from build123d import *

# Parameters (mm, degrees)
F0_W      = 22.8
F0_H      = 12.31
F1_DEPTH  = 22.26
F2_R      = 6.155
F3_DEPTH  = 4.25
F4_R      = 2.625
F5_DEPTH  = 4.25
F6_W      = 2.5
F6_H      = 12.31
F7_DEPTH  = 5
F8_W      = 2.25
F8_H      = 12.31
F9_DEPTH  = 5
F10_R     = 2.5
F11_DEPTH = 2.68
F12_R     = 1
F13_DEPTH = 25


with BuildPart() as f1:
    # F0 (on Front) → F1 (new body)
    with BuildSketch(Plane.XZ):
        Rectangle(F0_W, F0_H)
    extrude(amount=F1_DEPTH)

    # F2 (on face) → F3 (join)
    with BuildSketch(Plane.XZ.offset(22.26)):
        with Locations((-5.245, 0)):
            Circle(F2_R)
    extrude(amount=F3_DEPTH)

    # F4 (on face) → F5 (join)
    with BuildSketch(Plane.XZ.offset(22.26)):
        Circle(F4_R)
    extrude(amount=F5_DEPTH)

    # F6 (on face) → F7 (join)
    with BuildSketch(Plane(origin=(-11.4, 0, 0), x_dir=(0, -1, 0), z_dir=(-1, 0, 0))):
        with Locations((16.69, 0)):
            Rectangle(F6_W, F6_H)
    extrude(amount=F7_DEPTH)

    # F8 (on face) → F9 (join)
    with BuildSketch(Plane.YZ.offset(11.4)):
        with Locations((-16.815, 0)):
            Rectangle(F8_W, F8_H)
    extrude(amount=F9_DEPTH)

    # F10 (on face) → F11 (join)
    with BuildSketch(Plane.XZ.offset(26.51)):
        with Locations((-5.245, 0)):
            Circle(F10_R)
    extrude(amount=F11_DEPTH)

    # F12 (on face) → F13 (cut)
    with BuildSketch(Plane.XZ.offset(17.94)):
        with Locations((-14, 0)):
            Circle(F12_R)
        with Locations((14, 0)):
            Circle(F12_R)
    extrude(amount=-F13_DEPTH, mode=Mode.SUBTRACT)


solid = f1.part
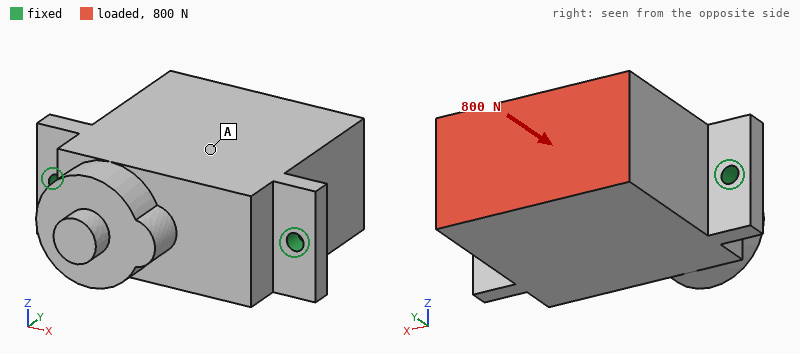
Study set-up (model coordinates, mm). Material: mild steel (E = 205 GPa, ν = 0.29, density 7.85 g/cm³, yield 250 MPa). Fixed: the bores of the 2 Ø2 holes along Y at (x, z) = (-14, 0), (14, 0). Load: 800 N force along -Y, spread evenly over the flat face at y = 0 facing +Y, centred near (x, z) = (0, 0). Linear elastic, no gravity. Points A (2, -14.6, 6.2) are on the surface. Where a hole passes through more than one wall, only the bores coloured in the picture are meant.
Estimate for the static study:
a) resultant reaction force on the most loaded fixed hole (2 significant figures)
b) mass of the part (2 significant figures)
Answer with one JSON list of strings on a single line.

["400 N", "56 g"]
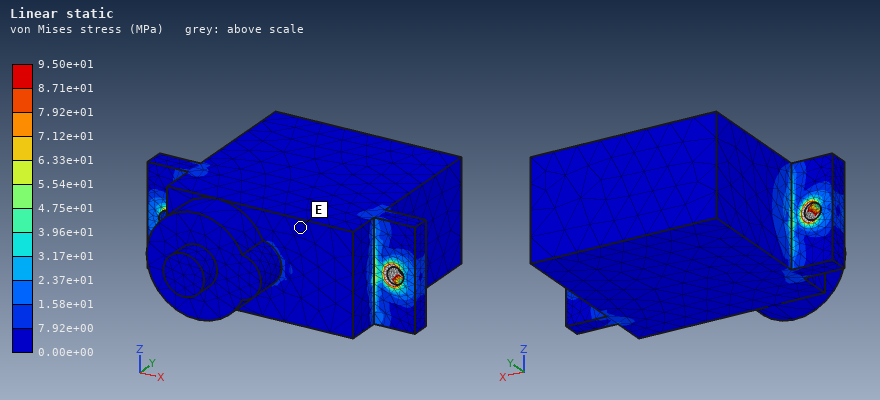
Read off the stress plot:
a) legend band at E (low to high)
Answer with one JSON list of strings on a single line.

["0.00e+00 to 7.92e+00 MPa"]
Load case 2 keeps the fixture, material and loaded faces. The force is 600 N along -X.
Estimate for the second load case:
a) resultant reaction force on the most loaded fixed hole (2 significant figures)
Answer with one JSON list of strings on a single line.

["510 N"]
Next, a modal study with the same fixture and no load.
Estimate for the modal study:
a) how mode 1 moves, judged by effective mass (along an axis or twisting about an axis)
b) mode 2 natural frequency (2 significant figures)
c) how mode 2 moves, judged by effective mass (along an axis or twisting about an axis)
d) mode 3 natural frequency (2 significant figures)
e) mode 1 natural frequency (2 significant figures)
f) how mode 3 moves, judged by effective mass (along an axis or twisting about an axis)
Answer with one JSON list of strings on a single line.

["along Z", "14 kHz", "along Y", "16 kHz", "3700 Hz", "along X"]
